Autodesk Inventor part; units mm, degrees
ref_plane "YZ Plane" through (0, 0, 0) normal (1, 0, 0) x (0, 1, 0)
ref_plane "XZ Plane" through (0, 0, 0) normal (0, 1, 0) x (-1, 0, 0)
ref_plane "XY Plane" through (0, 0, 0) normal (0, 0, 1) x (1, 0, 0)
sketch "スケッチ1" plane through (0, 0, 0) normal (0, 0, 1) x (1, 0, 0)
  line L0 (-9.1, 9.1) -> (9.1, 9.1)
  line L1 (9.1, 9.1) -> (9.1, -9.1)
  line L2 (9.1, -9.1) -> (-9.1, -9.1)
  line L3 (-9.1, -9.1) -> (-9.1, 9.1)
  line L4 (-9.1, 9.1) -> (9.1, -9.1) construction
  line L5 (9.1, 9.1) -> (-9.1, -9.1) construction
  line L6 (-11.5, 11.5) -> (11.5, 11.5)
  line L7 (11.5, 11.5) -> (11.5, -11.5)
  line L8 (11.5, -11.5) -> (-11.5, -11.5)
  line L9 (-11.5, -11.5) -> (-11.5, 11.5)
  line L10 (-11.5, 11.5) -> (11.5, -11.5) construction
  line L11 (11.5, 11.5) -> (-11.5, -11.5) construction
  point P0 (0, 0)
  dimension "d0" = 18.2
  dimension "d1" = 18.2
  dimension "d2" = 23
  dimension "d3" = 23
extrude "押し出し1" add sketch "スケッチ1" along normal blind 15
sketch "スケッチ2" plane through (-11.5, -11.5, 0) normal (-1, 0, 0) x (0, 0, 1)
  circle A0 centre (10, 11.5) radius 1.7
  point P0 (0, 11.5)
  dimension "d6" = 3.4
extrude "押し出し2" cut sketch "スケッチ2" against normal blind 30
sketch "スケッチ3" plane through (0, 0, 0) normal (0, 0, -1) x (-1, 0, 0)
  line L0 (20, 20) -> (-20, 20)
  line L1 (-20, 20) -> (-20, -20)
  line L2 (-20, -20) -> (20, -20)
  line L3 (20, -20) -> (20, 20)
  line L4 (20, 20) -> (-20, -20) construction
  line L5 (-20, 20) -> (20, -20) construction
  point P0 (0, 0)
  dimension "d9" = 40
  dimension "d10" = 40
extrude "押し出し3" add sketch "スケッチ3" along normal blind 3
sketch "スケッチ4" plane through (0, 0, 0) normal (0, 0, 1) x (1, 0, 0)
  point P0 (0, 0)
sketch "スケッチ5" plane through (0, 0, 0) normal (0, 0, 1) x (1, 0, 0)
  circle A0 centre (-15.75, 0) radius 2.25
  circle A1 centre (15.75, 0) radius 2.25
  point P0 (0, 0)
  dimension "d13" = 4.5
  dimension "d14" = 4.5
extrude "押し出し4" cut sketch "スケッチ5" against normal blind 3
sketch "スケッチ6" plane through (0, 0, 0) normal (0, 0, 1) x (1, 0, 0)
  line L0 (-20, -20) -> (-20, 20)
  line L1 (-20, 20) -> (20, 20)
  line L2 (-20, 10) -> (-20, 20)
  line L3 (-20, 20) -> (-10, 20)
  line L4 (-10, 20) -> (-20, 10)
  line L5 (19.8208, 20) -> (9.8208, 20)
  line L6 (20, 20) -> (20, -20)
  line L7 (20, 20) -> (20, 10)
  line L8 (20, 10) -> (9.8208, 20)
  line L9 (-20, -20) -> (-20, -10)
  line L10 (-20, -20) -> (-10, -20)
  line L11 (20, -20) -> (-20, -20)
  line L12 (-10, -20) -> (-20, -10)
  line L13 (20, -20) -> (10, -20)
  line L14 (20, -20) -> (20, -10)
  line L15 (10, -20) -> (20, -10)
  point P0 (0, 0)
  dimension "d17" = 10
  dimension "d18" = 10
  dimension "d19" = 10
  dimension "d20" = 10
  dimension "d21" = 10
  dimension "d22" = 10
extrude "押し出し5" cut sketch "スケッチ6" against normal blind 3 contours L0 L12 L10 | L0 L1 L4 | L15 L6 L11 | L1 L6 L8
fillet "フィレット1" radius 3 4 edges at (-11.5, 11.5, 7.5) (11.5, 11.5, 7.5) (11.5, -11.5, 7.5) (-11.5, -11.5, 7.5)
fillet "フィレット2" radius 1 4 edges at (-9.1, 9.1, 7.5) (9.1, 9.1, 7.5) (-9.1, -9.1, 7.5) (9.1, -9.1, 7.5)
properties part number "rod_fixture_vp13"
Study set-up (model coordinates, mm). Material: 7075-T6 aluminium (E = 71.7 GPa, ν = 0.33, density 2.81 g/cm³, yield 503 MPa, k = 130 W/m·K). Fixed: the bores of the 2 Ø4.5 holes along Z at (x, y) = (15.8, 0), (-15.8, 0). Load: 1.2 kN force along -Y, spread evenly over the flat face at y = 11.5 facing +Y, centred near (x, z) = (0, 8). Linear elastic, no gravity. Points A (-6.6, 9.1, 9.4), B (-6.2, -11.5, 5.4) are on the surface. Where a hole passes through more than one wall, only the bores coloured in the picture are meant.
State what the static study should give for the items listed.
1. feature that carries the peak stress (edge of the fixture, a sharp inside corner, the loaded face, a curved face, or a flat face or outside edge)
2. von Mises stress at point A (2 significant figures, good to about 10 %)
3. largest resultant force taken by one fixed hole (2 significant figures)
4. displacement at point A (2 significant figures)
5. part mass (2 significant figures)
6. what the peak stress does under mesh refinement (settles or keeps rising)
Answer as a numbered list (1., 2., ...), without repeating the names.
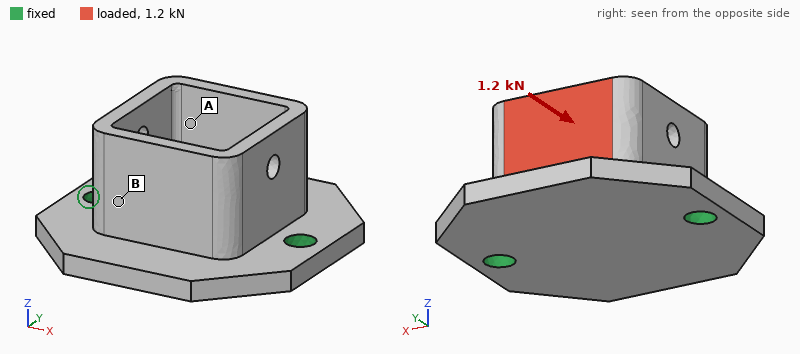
1. edge of the fixture
2. 41 MPa
3. 610 N
4. 0.073 mm
5. 19 g
6. keeps rising
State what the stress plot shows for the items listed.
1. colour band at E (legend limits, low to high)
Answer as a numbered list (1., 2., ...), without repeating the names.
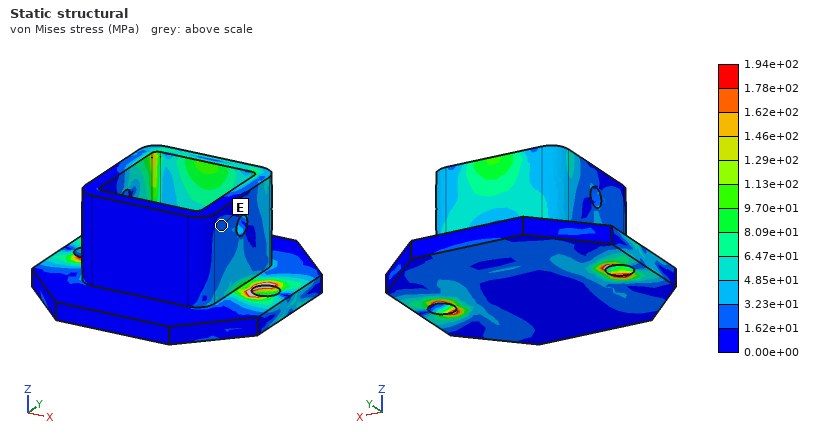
1. 1.62e+01 to 3.23e+01 MPa
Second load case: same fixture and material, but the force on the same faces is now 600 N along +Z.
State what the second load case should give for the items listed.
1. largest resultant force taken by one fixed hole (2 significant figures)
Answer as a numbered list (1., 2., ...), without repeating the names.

1. 310 N
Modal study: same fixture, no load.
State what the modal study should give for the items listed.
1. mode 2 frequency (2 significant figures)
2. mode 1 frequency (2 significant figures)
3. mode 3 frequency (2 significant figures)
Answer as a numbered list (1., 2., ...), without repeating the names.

1. 12 kHz
2. 5200 Hz
3. 13 kHz
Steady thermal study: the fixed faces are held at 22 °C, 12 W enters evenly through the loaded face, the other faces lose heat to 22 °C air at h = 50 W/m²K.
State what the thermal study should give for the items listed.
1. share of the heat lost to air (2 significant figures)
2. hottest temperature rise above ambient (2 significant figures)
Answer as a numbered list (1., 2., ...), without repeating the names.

1. 11 %
2. 16 K
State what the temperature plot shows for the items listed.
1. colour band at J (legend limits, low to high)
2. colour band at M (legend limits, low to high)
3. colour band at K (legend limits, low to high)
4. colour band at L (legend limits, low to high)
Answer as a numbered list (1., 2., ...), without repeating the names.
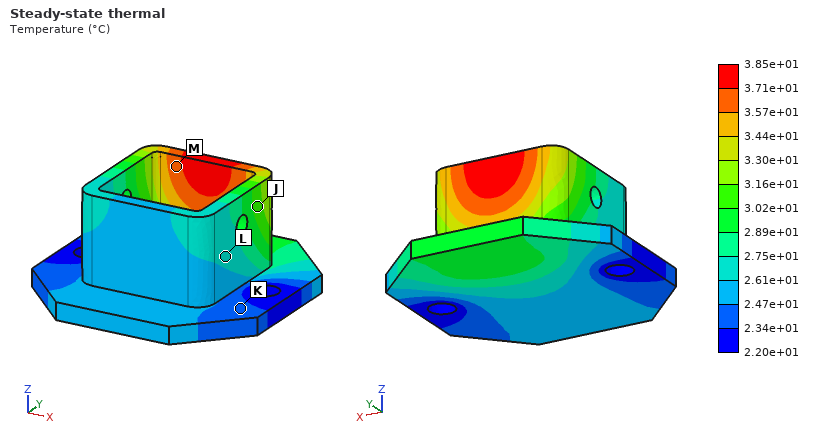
1. 3.02e+01 to 3.16e+01 °C
2. 3.57e+01 to 3.71e+01 °C
3. 2.34e+01 to 2.47e+01 °C
4. 2.61e+01 to 2.75e+01 °C
